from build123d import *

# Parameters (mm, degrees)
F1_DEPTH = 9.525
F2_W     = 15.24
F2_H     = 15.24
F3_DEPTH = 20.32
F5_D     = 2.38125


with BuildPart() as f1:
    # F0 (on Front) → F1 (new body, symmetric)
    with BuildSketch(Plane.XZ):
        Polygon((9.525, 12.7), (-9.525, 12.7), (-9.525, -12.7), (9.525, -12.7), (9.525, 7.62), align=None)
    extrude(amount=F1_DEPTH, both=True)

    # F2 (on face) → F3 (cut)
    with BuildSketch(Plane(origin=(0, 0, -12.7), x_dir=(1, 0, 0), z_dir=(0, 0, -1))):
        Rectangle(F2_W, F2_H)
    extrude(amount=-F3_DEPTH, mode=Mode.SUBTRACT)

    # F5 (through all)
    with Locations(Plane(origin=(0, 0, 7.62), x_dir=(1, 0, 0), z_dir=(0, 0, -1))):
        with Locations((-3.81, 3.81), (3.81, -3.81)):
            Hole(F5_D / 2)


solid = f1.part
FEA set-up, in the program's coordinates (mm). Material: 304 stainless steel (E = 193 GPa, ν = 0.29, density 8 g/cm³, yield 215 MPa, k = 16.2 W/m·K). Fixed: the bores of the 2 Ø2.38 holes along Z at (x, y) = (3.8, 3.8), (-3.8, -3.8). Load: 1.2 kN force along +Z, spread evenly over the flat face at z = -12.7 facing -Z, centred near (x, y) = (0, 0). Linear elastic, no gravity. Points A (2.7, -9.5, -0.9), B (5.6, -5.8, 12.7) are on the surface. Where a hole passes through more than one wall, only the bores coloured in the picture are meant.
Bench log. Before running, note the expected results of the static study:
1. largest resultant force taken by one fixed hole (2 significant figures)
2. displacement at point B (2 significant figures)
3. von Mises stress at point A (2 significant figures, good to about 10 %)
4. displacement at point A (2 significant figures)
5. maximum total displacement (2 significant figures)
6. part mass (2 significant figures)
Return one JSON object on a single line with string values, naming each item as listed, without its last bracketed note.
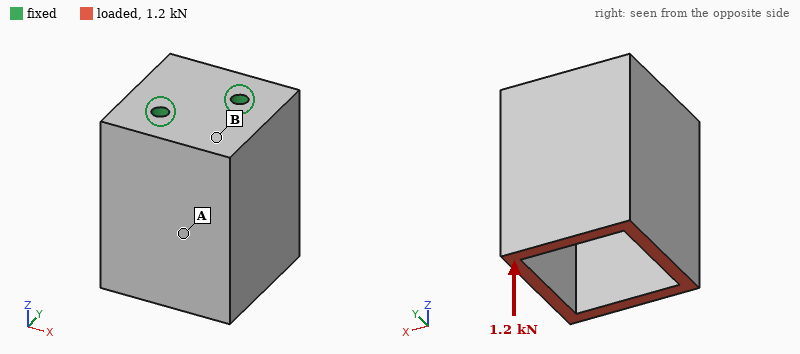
{"largest resultant force taken by one fixed hole": "600 N", "displacement at point B": "1.4 µm", "von Mises stress at point A": "12 MPa", "displacement at point A": "2.1 µm", "maximum total displacement": "3.7 µm", "part mass": "36 g"}
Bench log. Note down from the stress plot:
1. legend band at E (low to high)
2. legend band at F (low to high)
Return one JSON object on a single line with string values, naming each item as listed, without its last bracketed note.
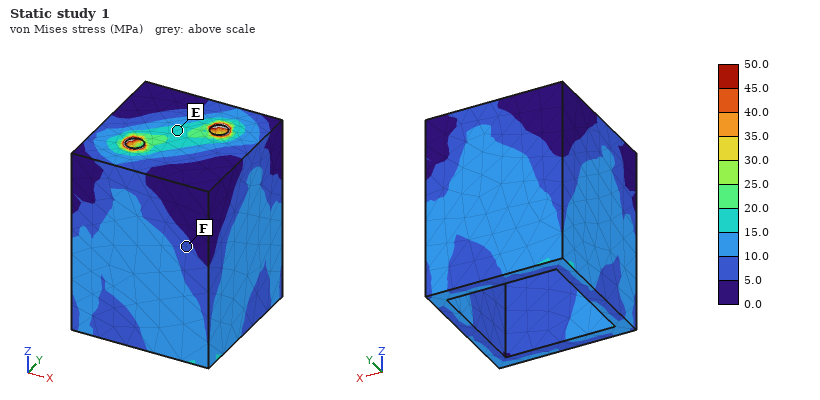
{"legend band at E": "15.0 to 20.0 MPa", "legend band at F": "5.0 to 10.0 MPa"}
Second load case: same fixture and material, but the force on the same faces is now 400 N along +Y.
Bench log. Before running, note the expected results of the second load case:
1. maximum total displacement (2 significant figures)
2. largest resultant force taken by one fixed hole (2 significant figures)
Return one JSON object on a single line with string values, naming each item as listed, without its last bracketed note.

{"maximum total displacement": "16 µm", "largest resultant force taken by one fixed hole": "460 N"}
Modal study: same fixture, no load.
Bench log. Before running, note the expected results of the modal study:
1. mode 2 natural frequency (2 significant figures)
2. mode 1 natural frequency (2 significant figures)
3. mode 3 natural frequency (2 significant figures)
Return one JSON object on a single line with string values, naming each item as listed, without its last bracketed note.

{"mode 2 natural frequency": "12 kHz", "mode 1 natural frequency": "8200 Hz", "mode 3 natural frequency": "13 kHz"}
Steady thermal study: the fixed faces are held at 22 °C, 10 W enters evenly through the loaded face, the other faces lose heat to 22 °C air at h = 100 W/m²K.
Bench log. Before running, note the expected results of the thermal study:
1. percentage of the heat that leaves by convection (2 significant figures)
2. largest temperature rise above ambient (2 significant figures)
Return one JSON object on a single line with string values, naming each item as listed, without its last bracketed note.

{"percentage of the heat that leaves by convection": "76 %", "largest temperature rise above ambient": "57 K"}
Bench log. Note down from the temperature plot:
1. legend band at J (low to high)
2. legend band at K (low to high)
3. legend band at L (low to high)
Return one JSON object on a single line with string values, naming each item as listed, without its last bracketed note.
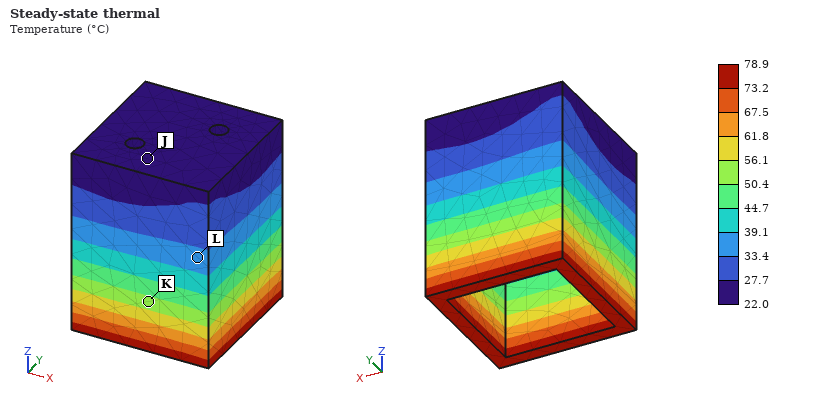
{"legend band at J": "22.0 to 27.7 °C", "legend band at K": "50.4 to 56.1 °C", "legend band at L": "33.4 to 39.1 °C"}
